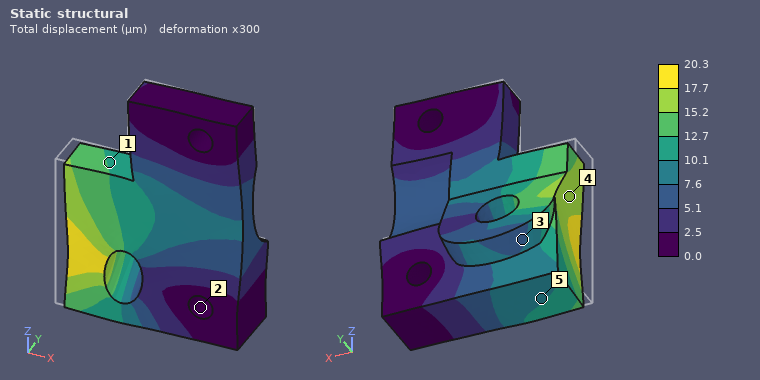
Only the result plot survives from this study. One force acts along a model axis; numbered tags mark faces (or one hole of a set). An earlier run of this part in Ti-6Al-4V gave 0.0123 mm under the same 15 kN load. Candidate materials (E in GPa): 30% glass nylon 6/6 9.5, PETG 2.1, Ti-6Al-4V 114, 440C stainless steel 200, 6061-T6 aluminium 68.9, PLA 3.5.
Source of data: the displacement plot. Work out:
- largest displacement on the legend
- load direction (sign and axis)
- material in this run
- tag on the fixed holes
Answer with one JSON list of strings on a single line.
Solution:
["20.3 µm", "+X", "6061-T6 aluminium", "2"]
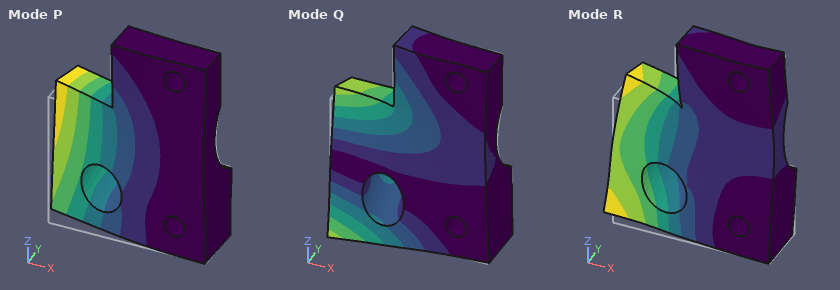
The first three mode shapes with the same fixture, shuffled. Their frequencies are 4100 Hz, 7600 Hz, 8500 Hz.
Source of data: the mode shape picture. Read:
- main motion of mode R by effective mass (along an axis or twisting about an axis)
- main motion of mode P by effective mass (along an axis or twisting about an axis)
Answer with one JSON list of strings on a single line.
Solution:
["along Z", "along Y"]
